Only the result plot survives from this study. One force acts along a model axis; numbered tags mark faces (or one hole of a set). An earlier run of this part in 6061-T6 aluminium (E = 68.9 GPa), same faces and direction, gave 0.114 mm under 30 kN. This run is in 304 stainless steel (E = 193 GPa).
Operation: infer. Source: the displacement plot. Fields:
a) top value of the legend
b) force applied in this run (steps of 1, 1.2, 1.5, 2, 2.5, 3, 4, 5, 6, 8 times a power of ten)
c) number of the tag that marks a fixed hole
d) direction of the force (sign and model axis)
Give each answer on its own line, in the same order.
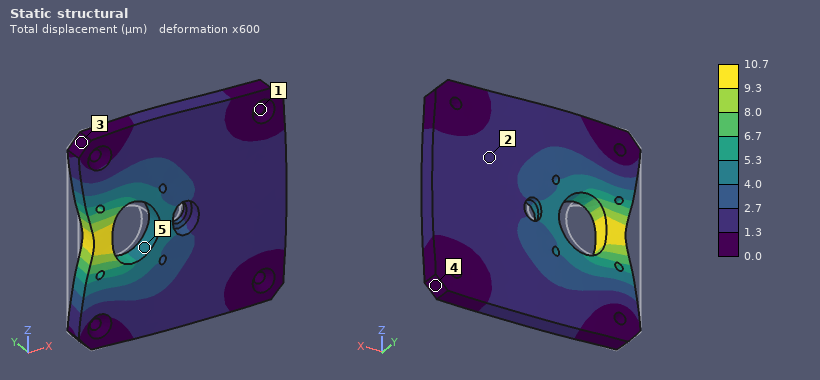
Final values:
10.7 µm
8 kN
1
+X
